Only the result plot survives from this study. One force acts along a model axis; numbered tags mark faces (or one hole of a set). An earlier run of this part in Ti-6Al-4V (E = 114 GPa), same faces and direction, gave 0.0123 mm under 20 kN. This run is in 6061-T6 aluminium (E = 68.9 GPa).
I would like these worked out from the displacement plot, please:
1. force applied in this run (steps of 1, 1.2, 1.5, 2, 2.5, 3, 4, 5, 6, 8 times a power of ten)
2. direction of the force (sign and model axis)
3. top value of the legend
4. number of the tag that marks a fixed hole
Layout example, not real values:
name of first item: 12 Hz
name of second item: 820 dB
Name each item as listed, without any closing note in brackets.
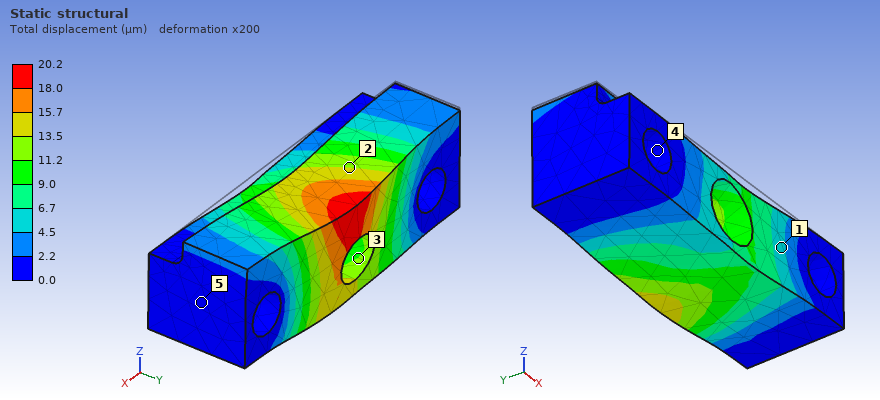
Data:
force applied in this run: 20 kN
direction of the force: -Z
top value of the legend: 20.2 µm
number of the tag that marks a fixed hole: 4
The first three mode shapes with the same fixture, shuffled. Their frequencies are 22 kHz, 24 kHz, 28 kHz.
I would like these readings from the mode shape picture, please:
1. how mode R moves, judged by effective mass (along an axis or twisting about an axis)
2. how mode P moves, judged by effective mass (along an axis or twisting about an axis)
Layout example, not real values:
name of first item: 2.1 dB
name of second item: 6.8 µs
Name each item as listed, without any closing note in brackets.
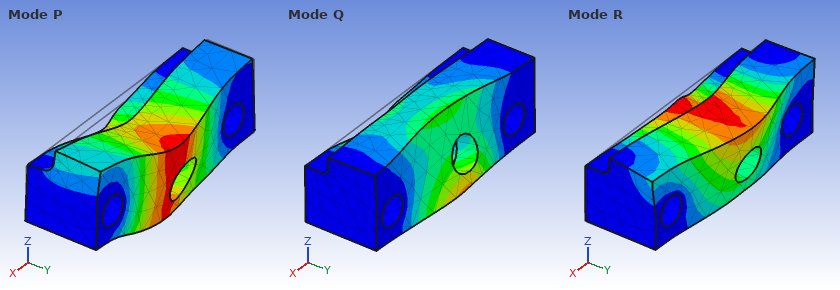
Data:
how mode R moves, judged by effective mass: along Y
how mode P moves, judged by effective mass: along Z
